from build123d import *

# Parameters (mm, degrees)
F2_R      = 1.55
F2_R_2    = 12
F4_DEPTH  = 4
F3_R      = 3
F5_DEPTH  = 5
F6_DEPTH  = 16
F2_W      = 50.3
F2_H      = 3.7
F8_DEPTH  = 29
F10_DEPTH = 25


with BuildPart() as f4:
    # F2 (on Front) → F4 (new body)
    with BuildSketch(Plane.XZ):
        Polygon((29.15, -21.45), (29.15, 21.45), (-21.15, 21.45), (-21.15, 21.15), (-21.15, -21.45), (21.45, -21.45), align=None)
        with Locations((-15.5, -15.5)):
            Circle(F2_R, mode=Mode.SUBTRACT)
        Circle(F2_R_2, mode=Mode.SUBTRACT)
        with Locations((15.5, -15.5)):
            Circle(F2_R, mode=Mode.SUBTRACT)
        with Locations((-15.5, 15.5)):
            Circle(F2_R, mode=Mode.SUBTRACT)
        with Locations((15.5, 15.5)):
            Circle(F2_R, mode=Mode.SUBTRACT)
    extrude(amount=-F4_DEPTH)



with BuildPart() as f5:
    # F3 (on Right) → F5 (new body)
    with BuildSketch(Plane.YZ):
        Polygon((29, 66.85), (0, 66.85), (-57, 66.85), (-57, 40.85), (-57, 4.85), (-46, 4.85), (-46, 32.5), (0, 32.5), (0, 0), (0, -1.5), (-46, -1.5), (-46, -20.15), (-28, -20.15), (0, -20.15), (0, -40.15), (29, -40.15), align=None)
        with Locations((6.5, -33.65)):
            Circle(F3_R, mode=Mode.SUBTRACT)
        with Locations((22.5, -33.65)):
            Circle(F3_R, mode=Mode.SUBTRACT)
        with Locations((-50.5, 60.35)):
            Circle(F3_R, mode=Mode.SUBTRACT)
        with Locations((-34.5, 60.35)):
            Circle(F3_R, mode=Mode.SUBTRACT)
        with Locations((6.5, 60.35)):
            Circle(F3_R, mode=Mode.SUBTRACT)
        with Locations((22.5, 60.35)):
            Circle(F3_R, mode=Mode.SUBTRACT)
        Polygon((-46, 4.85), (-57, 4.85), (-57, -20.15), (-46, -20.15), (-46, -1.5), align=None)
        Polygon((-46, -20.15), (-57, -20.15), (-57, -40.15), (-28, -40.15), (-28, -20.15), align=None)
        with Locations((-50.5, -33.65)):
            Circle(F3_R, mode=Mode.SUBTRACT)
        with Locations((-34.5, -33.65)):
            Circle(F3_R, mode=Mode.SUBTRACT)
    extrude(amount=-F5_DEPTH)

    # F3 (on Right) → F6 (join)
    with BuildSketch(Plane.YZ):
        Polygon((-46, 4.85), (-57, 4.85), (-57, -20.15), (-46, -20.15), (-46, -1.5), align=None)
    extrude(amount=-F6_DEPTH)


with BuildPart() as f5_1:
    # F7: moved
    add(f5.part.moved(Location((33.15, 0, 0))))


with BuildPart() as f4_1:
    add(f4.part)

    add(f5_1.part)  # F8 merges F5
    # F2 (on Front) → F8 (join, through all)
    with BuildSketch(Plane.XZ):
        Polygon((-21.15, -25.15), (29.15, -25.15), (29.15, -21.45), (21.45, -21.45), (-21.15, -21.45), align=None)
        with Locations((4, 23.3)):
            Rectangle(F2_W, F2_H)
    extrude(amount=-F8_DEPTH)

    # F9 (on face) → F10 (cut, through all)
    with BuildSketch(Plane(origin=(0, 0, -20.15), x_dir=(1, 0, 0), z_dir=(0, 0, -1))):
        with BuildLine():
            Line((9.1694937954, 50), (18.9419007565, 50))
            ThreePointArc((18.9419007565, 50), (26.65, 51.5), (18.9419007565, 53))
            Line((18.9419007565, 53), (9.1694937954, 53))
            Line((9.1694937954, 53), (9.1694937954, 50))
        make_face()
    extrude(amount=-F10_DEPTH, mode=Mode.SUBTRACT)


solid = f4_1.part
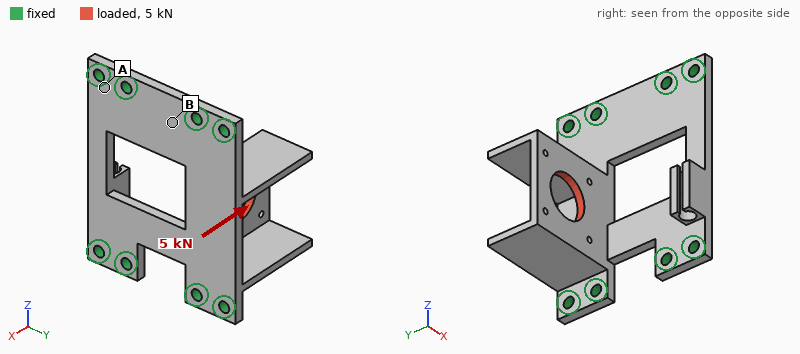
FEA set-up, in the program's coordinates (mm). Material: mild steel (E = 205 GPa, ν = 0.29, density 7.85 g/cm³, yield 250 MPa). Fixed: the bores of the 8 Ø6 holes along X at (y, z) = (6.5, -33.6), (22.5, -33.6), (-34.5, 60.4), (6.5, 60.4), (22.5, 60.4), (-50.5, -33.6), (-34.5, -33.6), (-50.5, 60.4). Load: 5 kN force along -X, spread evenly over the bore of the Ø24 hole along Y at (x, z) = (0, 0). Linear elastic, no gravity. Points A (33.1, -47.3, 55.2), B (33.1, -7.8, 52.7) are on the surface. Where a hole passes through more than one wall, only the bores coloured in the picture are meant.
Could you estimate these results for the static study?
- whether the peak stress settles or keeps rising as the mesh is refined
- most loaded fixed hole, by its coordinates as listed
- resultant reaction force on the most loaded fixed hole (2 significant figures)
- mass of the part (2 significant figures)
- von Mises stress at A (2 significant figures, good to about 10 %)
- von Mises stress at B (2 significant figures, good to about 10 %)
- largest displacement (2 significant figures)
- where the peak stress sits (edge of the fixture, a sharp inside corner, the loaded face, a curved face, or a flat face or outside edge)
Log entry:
keeps rising
(6.5, -33.6)
3.3 kN
420 g
31 MPa
69 MPa
0.19 mm
edge of the fixture
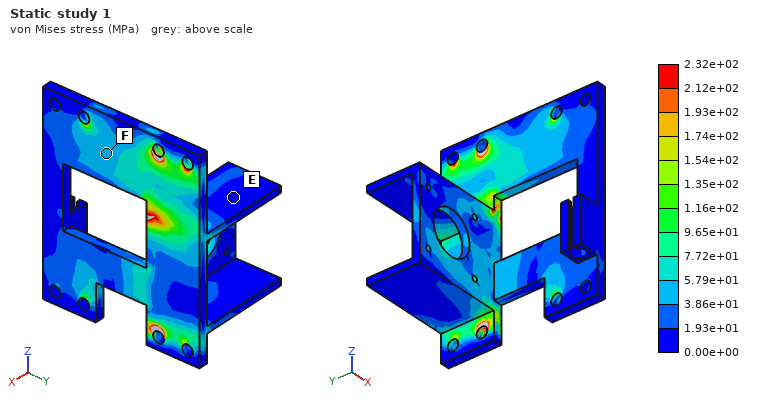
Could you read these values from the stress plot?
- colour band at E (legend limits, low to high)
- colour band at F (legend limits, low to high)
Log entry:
0.00e+00 to 1.93e+01 MPa
3.86e+01 to 5.79e+01 MPa
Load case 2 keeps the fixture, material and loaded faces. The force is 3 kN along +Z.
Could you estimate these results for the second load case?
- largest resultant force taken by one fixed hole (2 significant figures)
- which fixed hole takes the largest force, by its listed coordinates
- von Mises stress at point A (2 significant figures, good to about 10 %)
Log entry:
1.7 kN
(6.5, -33.6)
17 MPa
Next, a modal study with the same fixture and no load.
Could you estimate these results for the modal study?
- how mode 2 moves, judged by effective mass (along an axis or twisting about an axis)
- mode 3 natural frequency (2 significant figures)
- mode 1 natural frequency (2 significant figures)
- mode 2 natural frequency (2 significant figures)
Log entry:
along X
3300 Hz
1800 Hz
2200 Hz
